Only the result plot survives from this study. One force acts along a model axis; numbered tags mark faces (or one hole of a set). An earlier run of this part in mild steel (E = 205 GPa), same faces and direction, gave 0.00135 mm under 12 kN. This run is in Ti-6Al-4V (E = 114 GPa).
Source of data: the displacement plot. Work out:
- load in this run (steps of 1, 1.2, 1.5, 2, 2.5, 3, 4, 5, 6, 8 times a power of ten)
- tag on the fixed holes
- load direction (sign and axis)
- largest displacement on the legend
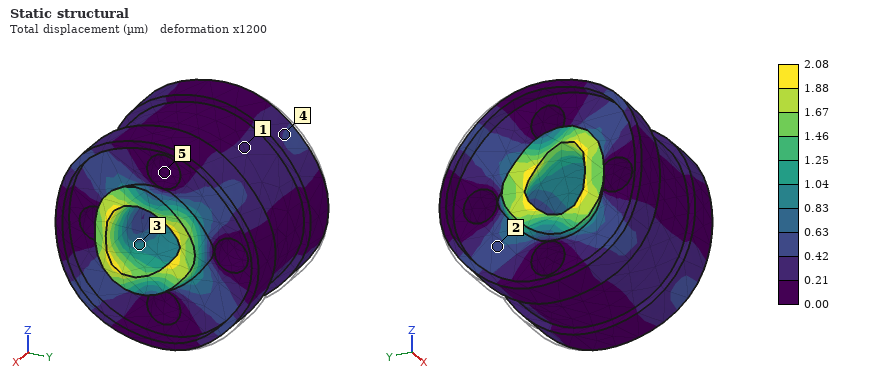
10 kN
5
-Y
2.08 µm
